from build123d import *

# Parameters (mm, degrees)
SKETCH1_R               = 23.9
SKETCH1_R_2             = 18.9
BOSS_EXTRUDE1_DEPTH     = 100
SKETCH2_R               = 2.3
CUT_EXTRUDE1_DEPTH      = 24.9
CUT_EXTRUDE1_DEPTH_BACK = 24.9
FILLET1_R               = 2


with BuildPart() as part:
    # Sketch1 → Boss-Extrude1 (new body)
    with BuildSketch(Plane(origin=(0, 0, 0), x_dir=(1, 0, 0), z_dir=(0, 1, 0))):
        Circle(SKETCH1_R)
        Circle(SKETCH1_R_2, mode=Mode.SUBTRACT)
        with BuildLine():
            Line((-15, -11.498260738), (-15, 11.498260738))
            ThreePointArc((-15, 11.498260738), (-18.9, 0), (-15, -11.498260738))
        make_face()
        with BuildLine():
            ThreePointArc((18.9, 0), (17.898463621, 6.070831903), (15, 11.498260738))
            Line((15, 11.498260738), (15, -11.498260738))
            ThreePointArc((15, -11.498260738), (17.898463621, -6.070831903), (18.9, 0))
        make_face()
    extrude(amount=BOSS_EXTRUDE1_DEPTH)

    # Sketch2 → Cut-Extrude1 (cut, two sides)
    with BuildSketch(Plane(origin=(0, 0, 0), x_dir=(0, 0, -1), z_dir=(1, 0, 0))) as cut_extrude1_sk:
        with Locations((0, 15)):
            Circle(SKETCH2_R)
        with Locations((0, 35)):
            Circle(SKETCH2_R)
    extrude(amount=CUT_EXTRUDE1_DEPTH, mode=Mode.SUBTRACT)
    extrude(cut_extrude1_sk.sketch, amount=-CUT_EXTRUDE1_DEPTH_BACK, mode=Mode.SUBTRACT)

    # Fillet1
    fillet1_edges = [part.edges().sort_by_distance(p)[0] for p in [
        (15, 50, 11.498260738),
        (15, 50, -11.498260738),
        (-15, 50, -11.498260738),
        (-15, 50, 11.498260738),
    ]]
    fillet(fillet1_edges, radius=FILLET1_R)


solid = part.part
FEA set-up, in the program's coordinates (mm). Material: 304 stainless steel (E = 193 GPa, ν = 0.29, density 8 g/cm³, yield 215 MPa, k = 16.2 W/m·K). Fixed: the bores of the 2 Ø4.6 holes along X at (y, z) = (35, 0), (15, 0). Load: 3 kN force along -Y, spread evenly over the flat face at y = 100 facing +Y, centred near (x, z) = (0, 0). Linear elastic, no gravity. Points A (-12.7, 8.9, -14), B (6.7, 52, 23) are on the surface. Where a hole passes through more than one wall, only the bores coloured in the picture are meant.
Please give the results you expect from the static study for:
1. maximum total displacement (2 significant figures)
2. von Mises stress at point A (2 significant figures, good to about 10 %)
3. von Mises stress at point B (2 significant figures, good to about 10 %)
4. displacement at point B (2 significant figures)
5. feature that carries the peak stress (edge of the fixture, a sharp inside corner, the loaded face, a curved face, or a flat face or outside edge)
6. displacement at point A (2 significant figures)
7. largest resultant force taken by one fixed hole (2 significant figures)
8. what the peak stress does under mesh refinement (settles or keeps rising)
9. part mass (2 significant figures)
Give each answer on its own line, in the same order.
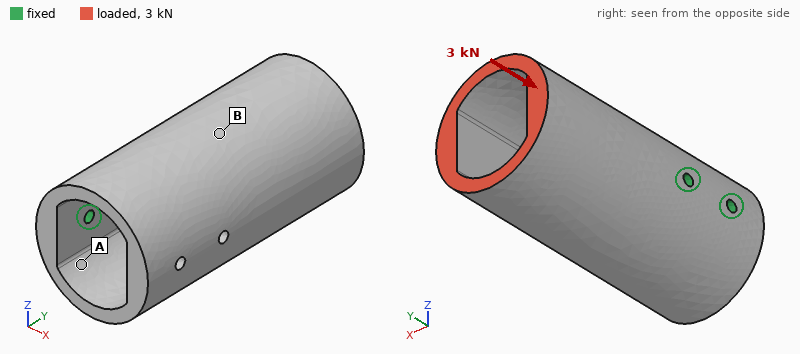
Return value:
34 µm
20 MPa
7.1 MPa
14 µm
edge of the fixture
5.5 µm
2.5 kN
keeps rising
630 g
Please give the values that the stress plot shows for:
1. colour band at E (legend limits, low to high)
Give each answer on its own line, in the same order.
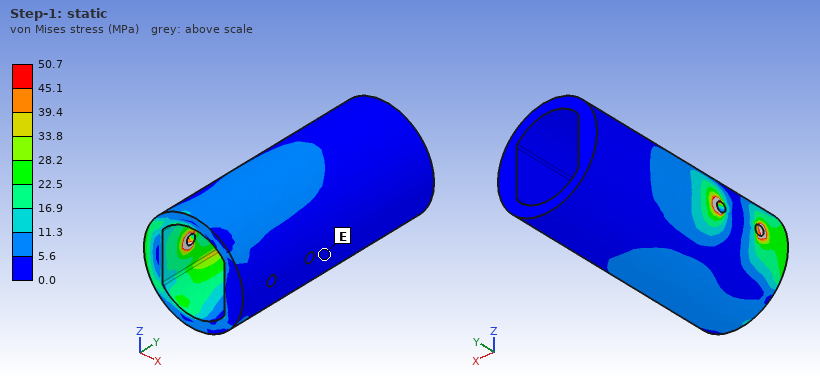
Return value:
0.0 to 5.6 MPa
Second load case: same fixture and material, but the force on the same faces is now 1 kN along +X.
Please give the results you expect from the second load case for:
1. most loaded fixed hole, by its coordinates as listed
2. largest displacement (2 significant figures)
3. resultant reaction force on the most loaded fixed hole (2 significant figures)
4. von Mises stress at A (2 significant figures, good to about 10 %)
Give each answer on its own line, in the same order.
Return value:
(35, 0)
49 µm
3.0 kN
23 MPa
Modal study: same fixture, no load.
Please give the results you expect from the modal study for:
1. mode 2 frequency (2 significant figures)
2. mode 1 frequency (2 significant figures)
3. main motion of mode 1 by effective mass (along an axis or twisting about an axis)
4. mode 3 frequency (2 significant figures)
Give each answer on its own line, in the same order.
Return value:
1700 Hz
1400 Hz
along Z
2900 Hz
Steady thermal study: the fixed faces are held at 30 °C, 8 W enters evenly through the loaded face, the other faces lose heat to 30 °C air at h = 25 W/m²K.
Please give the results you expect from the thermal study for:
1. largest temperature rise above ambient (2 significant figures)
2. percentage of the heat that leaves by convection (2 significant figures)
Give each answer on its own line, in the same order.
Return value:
27 K
78 %
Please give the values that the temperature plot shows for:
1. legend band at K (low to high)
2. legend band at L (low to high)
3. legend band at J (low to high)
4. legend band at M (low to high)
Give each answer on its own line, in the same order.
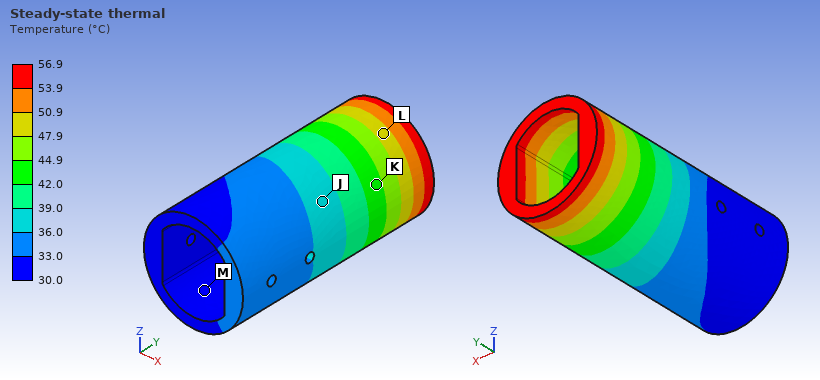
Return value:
42.0 to 44.9 °C
47.9 to 50.9 °C
36.0 to 39.0 °C
30.0 to 33.0 °C
